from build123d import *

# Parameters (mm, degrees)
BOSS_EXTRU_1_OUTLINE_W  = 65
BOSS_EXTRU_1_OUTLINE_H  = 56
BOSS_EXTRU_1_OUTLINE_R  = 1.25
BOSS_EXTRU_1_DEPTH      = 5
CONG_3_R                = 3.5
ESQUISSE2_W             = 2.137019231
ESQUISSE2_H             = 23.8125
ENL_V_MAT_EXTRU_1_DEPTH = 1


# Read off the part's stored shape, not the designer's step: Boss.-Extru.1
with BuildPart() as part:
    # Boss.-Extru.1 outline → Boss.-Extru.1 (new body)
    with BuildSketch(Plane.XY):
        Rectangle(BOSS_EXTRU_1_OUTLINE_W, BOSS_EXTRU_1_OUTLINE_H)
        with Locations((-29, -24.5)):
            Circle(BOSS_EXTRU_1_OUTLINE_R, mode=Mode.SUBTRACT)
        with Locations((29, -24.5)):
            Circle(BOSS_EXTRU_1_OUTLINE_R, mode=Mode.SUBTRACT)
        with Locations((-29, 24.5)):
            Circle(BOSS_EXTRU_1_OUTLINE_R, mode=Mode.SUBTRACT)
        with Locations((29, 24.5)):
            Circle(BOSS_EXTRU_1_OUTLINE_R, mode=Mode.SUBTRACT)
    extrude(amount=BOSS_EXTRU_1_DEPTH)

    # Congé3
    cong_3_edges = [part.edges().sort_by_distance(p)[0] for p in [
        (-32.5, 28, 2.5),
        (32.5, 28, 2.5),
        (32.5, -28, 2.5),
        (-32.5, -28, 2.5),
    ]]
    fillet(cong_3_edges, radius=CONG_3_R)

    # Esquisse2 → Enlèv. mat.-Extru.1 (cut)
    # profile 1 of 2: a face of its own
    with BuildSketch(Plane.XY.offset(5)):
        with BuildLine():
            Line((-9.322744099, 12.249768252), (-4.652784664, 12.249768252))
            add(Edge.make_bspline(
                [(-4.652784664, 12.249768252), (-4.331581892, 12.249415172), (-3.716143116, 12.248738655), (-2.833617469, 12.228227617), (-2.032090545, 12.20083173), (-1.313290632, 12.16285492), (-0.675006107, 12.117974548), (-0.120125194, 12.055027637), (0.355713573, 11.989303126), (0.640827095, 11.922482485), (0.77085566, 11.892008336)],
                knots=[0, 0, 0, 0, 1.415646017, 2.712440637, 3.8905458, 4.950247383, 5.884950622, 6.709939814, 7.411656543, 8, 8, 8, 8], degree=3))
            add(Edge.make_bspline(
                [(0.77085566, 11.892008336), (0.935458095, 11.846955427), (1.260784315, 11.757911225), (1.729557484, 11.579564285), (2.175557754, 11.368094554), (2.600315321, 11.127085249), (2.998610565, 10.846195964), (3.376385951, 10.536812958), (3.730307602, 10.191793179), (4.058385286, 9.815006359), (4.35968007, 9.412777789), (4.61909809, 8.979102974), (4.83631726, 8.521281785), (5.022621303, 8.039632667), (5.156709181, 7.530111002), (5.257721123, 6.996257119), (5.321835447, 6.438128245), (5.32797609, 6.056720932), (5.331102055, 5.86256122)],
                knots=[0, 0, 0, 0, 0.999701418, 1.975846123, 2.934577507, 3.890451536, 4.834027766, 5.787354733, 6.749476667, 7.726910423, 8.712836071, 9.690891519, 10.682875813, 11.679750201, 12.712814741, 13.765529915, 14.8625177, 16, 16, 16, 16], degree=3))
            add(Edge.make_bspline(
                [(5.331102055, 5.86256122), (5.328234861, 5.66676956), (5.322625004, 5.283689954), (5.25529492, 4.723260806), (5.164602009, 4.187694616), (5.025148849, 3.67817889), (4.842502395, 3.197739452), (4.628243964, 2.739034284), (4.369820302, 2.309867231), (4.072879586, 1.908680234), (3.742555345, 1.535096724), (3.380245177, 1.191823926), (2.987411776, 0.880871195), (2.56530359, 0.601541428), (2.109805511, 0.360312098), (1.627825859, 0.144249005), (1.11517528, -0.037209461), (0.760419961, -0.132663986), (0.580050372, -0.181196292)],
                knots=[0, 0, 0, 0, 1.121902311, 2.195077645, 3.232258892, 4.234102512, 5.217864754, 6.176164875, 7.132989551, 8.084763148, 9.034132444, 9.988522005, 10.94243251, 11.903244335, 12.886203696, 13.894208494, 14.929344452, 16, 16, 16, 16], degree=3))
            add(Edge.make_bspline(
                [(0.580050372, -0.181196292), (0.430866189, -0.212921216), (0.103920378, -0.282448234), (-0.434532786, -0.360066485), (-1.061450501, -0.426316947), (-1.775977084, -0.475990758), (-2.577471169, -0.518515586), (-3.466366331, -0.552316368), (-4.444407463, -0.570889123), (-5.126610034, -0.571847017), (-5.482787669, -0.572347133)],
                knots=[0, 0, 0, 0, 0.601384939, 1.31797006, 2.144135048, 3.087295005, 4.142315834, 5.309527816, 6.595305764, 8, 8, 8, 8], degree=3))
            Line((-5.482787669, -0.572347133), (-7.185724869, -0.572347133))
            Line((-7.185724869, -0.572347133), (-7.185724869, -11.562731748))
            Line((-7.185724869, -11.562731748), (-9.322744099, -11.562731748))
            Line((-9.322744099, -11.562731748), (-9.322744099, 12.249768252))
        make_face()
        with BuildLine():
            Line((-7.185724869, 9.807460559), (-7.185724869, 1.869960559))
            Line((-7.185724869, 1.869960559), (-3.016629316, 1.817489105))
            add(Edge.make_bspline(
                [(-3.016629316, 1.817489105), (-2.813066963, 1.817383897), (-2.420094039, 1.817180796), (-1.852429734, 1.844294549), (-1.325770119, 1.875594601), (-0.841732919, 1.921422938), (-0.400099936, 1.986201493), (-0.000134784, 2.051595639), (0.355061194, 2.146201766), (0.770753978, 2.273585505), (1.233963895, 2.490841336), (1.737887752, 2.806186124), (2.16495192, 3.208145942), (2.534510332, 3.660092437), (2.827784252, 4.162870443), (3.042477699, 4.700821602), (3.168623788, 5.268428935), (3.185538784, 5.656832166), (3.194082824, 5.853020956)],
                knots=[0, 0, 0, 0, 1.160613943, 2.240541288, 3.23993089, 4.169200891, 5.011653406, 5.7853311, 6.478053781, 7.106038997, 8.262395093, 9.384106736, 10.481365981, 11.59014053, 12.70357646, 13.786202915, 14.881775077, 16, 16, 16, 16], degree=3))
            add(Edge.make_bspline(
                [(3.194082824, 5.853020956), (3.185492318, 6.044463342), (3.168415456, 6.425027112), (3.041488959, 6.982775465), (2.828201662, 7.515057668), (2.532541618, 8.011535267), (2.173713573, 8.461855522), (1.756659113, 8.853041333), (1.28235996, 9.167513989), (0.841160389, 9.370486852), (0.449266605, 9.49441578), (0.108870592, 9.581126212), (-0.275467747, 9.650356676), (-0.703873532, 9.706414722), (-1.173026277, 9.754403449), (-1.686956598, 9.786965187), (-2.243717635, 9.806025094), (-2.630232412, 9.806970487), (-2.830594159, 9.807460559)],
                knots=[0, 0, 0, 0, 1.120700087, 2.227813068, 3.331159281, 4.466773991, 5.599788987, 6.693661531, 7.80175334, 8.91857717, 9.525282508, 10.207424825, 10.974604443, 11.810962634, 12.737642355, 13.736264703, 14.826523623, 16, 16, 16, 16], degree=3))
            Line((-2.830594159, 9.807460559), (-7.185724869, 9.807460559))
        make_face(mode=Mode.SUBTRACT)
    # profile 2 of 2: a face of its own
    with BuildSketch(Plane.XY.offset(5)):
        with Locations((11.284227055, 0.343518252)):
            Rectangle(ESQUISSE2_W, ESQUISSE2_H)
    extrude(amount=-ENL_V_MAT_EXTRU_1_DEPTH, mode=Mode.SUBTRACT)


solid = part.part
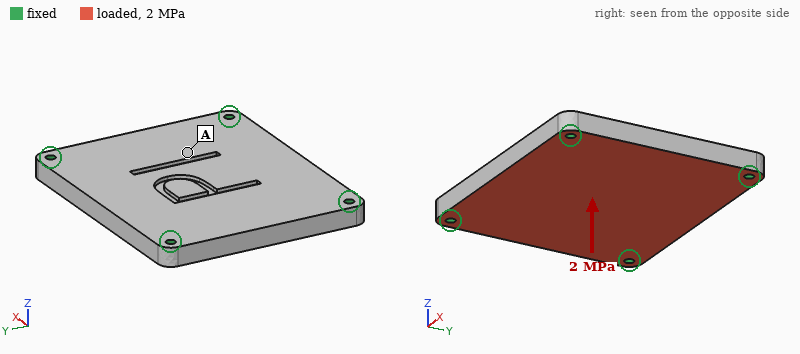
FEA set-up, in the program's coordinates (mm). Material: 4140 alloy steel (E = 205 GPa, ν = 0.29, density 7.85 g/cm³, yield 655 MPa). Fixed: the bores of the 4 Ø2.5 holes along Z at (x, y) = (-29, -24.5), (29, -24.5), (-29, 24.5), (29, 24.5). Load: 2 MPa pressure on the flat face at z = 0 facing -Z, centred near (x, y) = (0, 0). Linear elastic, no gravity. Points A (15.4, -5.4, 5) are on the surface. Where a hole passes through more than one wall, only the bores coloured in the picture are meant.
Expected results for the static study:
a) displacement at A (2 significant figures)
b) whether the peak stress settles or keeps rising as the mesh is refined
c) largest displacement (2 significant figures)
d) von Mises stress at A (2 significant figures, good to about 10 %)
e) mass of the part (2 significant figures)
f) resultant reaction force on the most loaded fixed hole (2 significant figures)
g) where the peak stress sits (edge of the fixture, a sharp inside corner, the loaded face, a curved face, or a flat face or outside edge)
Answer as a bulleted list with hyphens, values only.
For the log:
- 57 µm
- keeps rising
- 76 µm
- 65 MPa
- 140 g
- 1.8 kN
- edge of the fixture
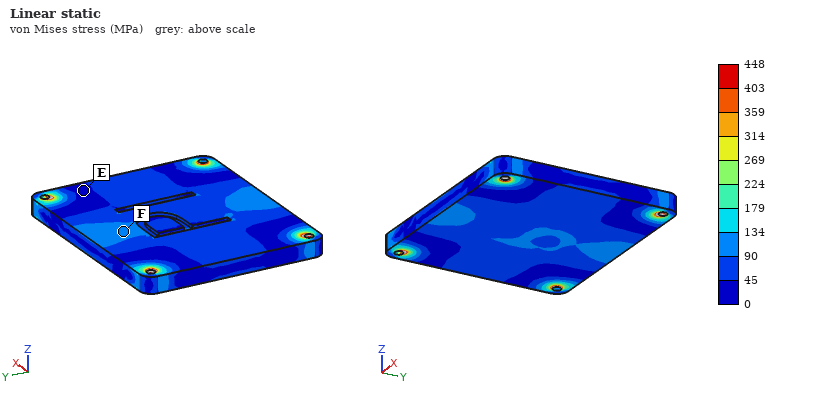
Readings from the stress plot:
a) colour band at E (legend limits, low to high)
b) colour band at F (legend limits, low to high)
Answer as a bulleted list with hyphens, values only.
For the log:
- 0 to 45 MPa
- 90 to 134 MPa
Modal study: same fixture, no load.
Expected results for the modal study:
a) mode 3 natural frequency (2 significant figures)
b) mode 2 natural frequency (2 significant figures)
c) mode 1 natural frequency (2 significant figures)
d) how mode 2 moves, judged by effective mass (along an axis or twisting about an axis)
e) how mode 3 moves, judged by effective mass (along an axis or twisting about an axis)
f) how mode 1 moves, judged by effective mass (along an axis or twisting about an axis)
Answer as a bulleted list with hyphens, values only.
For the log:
- 9900 Hz
- 8300 Hz
- 5000 Hz
- twisting about X
- twisting about Y
- along Z
